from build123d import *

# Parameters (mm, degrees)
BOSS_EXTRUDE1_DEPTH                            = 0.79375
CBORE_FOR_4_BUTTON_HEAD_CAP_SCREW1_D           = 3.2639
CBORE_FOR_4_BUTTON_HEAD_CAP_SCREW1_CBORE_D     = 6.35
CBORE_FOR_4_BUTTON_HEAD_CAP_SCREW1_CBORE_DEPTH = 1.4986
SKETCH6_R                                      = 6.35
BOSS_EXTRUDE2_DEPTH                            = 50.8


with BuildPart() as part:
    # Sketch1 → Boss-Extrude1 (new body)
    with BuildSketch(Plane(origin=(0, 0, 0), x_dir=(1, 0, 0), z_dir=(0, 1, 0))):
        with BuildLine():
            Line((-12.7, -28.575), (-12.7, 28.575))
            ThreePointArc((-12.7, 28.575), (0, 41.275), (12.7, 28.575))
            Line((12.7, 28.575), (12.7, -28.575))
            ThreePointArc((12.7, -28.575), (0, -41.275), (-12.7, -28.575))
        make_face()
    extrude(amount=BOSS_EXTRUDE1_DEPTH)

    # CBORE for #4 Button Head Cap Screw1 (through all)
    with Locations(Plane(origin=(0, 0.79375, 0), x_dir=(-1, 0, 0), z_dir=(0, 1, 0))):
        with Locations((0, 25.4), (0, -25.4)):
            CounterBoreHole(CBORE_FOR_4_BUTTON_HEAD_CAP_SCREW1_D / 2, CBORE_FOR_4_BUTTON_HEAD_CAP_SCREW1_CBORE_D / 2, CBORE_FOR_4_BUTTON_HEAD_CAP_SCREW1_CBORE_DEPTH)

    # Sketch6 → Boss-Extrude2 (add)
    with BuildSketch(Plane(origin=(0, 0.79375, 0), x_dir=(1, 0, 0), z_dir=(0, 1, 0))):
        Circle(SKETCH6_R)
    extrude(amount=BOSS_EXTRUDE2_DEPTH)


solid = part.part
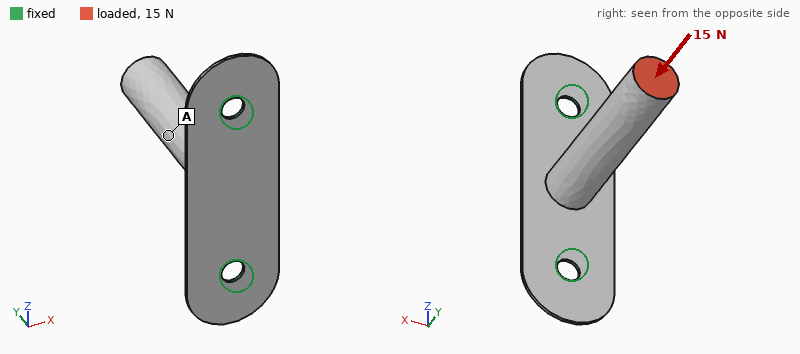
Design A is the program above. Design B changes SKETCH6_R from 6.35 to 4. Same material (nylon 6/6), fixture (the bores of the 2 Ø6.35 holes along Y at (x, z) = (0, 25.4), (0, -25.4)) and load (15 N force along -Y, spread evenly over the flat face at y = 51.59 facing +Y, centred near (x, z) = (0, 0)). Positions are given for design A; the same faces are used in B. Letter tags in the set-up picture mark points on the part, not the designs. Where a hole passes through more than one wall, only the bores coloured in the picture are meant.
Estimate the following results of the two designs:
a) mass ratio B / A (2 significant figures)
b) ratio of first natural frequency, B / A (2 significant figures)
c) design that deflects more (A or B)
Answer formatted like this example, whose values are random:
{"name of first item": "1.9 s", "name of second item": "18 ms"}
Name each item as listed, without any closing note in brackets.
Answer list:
{"mass ratio B / A": "0.51", "ratio of first natural frequency, B / A": "1.4", "design that deflects more": "B"}
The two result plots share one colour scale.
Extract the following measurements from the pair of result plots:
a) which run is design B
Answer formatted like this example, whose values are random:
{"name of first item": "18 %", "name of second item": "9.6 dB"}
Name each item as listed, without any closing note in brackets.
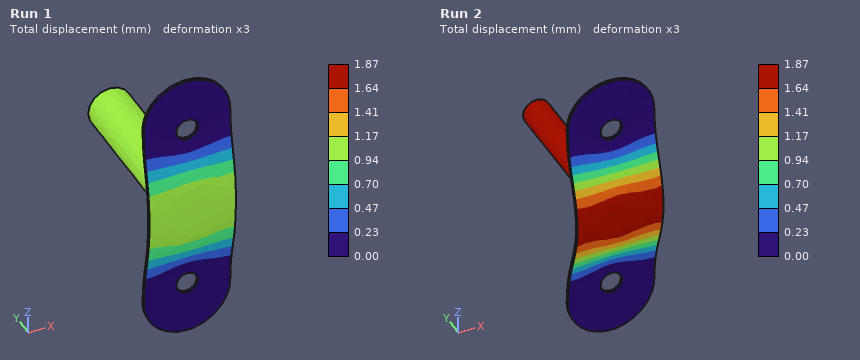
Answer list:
{"which run is design B": "Run 2"}
